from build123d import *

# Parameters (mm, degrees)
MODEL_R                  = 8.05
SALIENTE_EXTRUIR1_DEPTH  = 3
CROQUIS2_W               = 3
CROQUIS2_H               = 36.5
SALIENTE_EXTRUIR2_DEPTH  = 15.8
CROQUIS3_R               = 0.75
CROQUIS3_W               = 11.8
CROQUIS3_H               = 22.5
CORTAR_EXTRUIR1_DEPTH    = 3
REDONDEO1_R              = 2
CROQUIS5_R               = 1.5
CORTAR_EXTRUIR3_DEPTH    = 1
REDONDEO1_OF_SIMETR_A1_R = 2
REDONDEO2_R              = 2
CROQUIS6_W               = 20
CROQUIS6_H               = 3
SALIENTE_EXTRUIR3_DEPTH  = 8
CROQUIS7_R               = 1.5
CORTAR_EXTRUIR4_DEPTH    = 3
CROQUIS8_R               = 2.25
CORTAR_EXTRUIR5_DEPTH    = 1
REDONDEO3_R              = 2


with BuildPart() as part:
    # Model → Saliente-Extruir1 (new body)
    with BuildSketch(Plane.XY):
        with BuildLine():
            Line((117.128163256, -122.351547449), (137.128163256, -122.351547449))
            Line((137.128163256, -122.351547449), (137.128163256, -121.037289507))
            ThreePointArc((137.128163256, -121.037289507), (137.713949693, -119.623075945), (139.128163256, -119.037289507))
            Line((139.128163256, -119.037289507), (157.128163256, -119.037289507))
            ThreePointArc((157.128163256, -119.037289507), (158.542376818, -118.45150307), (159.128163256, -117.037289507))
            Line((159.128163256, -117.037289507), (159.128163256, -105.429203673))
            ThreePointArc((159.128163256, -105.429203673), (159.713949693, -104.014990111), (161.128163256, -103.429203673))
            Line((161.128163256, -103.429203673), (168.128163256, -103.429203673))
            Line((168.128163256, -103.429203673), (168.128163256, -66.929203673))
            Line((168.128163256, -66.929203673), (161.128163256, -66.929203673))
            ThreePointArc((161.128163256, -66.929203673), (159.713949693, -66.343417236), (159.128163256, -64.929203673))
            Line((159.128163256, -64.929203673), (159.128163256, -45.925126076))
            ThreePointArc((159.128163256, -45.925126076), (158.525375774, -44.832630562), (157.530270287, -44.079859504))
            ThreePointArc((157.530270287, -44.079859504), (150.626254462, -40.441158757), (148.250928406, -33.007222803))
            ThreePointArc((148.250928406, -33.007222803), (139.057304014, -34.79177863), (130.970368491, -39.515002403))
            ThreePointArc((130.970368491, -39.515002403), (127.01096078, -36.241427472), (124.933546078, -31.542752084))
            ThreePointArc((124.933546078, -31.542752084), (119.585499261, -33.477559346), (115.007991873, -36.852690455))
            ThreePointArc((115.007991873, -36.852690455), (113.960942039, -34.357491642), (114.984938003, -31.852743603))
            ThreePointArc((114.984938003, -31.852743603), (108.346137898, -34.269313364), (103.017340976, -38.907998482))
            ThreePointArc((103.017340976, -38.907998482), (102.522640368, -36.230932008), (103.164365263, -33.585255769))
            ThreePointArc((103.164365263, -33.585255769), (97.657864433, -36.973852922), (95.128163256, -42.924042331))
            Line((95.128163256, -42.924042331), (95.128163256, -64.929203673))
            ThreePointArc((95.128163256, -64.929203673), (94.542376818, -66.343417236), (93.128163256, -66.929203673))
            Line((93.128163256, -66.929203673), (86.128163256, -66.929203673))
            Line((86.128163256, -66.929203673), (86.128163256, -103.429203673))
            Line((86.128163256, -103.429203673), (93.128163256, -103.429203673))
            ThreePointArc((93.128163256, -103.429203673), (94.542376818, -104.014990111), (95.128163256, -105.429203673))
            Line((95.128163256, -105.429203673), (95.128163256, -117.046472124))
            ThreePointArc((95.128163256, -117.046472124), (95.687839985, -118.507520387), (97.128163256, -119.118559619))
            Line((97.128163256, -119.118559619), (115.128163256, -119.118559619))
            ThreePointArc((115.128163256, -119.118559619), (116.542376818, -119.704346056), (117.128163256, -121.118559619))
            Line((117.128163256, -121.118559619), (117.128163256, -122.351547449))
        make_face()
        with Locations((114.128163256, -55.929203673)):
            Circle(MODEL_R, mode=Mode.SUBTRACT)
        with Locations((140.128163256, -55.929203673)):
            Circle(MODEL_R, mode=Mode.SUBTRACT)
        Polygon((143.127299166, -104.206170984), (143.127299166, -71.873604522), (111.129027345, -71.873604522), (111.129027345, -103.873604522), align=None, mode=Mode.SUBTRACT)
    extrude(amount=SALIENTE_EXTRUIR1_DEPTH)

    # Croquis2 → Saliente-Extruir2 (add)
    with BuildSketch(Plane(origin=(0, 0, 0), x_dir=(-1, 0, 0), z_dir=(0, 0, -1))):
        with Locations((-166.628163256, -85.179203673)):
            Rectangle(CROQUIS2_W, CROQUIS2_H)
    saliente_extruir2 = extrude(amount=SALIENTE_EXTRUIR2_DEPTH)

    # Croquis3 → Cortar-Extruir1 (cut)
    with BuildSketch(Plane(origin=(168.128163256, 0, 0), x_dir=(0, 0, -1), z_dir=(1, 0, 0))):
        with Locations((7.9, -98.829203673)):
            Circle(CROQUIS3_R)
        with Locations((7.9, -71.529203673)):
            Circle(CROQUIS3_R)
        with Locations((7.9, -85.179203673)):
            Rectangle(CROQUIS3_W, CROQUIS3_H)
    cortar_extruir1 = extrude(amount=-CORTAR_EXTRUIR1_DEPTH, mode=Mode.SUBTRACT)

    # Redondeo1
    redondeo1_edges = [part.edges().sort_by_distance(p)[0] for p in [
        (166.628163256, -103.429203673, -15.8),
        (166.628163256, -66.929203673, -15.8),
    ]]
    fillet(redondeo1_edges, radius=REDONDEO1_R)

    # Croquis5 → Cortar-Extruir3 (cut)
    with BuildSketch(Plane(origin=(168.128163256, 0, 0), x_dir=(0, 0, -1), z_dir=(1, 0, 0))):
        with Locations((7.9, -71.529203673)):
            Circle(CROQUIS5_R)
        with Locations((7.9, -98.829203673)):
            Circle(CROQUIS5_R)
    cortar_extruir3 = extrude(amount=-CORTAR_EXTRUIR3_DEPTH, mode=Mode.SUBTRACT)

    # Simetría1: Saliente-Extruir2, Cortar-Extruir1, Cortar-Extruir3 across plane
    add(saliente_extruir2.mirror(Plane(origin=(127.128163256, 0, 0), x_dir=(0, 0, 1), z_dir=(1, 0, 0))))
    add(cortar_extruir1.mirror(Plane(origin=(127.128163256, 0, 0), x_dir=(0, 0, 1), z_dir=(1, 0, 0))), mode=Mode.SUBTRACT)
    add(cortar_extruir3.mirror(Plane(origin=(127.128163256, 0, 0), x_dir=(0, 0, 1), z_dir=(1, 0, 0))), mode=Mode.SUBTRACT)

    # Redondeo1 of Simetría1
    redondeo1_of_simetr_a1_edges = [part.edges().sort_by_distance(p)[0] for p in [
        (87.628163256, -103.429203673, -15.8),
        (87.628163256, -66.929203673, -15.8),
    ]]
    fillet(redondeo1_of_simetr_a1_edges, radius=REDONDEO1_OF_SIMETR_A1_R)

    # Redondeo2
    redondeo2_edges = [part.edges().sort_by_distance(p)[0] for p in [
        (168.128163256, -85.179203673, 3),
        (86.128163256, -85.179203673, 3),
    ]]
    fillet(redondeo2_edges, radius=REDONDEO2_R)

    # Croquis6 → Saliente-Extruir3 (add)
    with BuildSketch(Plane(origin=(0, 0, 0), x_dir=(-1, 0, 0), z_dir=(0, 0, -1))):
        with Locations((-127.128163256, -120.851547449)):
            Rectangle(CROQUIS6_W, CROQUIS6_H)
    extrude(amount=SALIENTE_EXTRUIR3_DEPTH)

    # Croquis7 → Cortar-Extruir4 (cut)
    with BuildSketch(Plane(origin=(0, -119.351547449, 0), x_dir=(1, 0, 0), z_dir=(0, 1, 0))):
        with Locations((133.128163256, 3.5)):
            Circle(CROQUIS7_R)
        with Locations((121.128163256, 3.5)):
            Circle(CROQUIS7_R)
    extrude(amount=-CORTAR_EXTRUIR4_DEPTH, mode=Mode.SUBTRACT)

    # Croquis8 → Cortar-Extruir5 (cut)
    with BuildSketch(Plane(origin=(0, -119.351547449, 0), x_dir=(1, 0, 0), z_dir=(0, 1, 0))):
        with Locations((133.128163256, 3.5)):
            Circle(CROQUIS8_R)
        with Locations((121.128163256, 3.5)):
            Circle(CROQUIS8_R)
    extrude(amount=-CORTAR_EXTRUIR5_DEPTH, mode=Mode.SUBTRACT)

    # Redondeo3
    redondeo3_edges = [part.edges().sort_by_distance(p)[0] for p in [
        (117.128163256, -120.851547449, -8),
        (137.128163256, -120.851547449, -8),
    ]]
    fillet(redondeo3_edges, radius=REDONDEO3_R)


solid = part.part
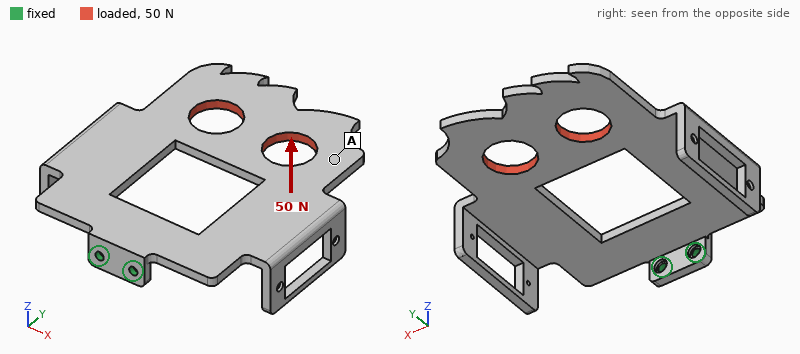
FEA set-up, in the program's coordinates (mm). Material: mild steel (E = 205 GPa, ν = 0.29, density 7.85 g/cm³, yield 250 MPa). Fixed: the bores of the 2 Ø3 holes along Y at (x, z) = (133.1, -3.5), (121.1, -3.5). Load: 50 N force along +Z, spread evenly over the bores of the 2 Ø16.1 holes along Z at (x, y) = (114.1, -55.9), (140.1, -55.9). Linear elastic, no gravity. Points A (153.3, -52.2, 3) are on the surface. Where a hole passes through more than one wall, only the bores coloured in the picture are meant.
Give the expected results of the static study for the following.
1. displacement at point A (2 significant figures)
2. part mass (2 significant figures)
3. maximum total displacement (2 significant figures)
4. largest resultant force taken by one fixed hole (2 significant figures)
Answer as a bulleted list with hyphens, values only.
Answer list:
- 0.48 mm
- 120 g
- 0.66 mm
- 51 N
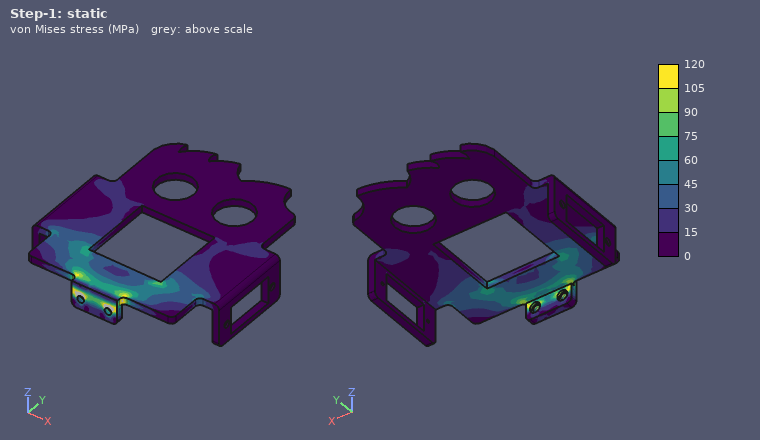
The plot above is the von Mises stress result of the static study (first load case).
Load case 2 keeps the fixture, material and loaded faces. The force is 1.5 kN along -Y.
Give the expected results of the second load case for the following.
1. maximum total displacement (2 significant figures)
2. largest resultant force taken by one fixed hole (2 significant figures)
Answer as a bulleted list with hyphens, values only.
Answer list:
- 0.26 mm
- 760 N
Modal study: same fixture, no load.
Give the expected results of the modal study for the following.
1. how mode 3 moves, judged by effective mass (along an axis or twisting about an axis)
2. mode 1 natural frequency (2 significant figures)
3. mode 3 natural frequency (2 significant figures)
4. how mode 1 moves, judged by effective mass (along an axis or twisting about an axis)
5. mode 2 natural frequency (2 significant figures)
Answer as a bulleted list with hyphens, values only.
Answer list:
- along X
- 210 Hz
- 780 Hz
- along Z
- 470 Hz
